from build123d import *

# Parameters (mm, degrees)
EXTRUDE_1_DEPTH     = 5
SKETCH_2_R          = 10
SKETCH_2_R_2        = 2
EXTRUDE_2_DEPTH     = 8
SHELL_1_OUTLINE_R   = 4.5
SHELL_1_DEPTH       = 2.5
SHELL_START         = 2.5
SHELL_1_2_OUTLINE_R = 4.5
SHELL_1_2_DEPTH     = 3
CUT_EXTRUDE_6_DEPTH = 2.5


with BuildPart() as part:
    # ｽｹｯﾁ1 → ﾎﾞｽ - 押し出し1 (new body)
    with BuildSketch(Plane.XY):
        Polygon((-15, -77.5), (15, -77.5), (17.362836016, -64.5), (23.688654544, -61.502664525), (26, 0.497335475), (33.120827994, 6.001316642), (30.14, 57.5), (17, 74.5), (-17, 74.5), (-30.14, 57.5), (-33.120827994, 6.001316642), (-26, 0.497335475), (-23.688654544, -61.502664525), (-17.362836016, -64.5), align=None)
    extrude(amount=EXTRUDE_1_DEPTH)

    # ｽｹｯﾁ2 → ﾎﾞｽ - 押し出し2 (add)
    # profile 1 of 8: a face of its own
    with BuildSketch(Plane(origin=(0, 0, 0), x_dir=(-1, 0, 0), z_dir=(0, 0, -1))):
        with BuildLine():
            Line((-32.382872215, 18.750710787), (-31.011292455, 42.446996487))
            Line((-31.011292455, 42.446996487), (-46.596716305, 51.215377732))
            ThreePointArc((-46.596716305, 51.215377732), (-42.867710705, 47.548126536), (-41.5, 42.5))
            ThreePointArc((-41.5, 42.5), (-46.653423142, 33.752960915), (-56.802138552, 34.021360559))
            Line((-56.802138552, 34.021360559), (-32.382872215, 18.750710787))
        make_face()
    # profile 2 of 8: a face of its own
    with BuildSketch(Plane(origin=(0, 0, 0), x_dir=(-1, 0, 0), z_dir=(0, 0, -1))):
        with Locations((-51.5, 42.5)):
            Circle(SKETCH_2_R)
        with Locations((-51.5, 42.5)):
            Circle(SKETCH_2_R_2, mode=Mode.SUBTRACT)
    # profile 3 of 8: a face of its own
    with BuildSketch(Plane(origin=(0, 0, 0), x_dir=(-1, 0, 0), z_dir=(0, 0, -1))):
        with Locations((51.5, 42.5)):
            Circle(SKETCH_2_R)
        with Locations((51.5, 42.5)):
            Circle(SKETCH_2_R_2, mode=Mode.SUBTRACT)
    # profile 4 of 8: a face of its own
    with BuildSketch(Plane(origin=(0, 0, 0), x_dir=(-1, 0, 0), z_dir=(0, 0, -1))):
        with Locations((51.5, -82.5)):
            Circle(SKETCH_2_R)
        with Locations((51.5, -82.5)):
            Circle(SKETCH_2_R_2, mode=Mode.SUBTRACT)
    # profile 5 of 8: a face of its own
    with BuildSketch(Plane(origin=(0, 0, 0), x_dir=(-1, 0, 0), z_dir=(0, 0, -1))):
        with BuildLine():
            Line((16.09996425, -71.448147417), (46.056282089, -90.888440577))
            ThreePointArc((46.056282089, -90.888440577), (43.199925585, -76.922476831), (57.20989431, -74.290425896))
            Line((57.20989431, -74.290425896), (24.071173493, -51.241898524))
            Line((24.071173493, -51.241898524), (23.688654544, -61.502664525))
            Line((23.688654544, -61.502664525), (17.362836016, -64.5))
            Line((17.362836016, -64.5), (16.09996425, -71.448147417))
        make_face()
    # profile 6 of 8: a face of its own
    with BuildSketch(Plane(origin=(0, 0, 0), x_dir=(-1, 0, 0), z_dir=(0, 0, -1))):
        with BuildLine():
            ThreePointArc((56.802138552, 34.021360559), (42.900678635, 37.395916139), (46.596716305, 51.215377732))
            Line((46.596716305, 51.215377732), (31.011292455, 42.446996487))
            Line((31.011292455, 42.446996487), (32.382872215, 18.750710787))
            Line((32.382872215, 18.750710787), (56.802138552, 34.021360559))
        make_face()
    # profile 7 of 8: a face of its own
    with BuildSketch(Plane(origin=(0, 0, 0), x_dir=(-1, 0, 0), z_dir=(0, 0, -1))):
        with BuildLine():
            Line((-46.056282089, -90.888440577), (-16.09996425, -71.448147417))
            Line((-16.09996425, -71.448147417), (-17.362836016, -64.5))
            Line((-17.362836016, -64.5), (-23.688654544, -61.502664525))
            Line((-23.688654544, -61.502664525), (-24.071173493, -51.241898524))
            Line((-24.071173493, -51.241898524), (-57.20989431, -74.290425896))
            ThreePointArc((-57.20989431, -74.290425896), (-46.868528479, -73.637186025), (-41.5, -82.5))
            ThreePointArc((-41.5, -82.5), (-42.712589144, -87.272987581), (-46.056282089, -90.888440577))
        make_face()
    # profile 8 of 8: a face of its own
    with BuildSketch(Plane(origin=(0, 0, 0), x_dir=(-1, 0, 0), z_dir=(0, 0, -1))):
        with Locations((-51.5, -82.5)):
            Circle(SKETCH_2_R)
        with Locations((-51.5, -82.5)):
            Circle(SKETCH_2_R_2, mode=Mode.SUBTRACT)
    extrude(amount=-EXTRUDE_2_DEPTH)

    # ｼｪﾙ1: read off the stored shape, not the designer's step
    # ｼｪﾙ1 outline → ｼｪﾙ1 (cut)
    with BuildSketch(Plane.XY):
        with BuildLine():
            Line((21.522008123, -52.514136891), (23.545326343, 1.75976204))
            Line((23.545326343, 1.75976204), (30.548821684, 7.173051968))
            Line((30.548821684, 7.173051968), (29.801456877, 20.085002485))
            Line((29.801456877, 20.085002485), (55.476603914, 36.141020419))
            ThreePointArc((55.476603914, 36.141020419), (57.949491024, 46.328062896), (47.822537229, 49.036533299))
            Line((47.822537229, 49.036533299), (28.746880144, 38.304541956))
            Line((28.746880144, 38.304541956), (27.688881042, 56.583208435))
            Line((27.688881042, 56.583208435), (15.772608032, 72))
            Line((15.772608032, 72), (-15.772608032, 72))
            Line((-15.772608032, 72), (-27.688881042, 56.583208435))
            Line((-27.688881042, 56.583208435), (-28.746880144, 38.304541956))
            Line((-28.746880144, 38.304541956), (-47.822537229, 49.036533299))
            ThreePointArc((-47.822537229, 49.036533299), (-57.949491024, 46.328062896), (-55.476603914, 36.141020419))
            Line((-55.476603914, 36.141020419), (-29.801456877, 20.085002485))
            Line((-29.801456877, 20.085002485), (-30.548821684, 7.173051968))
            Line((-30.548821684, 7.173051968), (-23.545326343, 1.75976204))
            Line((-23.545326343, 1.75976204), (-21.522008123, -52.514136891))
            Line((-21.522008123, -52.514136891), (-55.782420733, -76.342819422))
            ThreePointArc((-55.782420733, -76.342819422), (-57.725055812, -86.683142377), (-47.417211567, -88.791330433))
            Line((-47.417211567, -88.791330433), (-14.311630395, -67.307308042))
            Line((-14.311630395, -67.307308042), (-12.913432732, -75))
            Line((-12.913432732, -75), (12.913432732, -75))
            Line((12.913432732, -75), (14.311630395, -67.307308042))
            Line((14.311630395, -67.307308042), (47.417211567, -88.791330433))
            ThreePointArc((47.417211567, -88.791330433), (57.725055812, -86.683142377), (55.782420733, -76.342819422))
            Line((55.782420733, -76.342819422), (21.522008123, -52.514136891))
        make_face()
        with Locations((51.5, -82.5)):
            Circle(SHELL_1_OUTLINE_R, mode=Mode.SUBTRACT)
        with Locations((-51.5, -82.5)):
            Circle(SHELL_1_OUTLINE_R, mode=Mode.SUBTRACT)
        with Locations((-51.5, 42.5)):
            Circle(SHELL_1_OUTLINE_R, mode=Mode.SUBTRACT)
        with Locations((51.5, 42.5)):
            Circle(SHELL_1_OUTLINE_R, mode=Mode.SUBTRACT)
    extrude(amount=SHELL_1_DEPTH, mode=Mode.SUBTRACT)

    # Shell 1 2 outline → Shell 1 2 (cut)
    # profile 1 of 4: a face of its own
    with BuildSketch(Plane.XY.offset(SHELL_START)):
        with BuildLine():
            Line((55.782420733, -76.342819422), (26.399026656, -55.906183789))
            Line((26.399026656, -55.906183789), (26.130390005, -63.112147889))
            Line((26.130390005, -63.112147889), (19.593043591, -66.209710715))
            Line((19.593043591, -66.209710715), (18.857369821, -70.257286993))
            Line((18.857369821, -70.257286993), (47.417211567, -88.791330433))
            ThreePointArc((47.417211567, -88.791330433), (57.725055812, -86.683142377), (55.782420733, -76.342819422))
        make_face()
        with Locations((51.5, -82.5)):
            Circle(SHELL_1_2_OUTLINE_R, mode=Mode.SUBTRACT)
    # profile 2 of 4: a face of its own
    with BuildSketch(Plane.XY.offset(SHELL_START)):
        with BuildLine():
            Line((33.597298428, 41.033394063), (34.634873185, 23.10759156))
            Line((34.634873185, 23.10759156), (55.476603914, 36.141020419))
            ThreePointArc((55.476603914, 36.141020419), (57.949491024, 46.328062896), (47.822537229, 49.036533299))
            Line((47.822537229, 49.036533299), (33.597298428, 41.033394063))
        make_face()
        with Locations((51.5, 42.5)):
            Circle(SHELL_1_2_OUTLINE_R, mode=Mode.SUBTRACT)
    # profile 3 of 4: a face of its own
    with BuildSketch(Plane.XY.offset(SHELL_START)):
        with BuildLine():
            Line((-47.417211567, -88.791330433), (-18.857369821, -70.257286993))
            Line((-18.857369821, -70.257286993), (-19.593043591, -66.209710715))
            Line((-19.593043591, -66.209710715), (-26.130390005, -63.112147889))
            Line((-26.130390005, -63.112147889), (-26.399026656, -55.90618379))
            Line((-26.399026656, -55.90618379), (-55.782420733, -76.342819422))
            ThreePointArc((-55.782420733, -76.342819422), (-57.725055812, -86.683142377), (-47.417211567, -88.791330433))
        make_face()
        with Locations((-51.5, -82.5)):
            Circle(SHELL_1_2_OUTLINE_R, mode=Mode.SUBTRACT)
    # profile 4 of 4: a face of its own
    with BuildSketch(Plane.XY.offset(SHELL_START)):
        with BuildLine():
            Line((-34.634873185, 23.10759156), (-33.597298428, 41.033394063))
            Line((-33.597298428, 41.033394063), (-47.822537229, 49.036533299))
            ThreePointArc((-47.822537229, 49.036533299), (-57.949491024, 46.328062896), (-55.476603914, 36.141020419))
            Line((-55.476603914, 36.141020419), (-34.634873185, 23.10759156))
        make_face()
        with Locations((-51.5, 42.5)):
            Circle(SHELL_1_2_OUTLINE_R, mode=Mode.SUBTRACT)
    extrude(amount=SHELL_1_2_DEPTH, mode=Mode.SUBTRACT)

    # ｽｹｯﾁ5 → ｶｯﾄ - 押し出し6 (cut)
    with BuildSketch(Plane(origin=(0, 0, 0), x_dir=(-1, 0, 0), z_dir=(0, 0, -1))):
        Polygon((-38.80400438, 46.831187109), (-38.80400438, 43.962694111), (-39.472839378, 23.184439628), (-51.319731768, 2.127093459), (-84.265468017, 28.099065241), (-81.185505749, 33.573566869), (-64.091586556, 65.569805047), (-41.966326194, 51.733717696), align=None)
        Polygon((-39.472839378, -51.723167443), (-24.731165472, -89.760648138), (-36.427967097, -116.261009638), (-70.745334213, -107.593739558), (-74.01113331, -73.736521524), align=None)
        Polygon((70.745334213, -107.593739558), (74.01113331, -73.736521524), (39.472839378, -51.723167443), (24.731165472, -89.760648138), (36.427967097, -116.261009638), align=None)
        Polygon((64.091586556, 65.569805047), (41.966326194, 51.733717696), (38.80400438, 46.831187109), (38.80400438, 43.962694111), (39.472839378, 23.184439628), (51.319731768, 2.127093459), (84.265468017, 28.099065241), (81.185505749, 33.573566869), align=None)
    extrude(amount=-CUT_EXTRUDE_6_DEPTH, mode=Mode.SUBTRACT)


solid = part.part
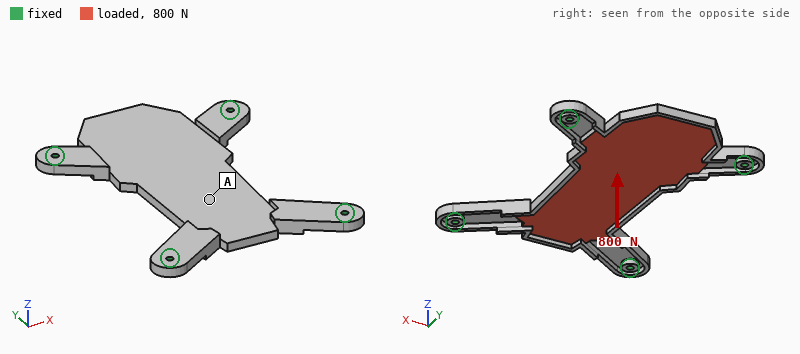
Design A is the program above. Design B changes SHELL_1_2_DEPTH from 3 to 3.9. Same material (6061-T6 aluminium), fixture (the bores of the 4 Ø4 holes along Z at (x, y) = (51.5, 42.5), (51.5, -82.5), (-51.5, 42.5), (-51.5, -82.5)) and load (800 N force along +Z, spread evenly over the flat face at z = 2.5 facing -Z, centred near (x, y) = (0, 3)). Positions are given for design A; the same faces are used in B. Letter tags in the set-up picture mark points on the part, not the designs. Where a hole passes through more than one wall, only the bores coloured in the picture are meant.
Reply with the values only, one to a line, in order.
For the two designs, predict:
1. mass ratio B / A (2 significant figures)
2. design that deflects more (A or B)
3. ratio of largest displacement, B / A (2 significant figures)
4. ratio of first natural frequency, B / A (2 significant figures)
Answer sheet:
0.95
B
1.1
0.94
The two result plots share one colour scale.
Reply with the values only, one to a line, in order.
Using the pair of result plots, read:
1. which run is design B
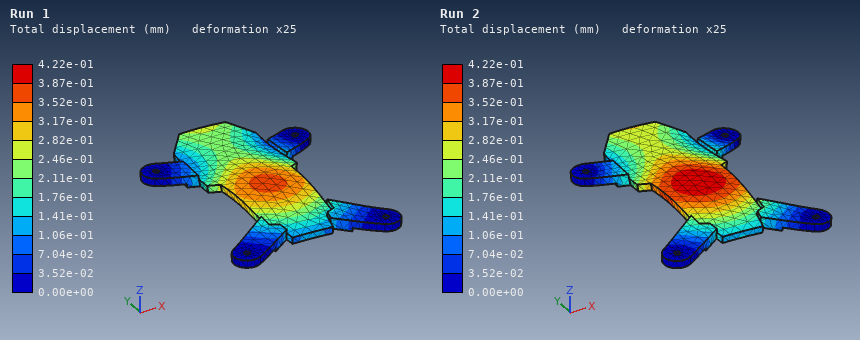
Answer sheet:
Run 2
